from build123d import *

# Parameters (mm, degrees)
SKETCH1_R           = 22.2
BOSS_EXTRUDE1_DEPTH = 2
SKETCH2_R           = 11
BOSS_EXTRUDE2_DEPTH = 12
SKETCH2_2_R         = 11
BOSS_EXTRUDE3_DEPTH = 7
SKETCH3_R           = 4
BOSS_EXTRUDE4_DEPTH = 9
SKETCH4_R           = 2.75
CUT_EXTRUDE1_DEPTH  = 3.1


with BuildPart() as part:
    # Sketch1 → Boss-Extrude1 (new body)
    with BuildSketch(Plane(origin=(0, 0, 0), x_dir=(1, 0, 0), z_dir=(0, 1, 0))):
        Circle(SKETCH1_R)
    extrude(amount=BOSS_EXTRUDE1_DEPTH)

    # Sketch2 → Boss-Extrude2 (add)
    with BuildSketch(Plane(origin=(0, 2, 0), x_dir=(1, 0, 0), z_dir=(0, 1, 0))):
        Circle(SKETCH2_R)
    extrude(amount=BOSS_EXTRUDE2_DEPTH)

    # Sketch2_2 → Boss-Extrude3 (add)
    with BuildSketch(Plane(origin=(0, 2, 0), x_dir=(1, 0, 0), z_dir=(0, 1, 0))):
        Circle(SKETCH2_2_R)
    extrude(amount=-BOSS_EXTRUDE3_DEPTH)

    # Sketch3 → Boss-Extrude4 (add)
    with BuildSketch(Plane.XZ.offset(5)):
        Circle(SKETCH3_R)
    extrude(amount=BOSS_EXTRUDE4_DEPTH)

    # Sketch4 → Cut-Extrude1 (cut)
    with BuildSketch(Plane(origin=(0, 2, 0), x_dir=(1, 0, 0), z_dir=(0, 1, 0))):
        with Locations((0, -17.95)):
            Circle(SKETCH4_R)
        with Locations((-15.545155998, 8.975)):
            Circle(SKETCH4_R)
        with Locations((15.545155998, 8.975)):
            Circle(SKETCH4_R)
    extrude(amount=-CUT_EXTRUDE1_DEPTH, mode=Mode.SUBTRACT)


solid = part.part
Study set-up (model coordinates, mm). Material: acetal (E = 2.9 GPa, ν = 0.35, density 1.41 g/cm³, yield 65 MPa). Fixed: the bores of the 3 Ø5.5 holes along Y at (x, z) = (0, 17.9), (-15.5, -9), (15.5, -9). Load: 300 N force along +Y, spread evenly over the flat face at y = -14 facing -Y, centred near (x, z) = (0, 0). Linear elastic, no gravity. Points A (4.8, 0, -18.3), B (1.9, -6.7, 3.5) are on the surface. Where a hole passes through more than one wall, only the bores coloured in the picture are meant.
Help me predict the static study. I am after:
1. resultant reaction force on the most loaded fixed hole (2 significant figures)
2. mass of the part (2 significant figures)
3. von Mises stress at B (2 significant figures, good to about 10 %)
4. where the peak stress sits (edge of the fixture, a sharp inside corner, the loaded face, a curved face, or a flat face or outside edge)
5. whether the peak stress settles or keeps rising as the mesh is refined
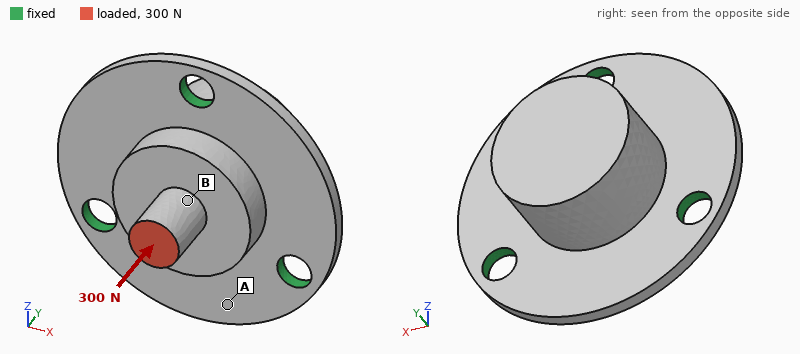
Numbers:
100 N
14 g
6.3 MPa
edge of the fixture
keeps rising
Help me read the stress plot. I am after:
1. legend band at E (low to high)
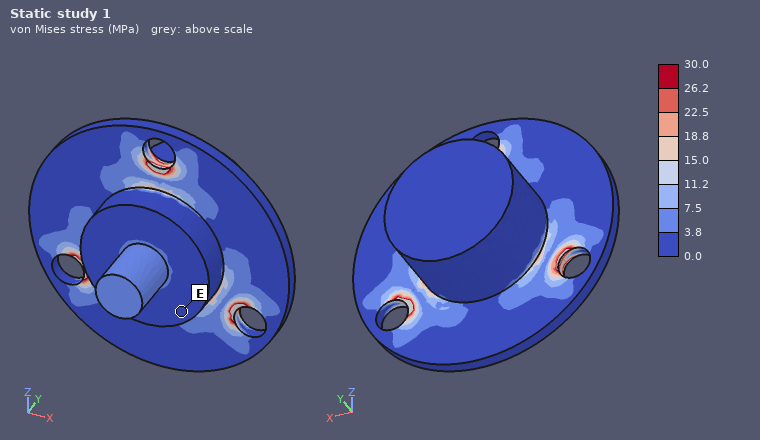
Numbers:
0.0 to 3.8 MPa
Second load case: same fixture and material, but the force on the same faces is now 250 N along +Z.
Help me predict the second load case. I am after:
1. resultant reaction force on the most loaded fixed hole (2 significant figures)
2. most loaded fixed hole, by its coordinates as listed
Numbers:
200 N
(0, 17.9)
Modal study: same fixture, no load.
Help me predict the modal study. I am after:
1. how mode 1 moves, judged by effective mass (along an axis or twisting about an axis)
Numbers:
along Y
